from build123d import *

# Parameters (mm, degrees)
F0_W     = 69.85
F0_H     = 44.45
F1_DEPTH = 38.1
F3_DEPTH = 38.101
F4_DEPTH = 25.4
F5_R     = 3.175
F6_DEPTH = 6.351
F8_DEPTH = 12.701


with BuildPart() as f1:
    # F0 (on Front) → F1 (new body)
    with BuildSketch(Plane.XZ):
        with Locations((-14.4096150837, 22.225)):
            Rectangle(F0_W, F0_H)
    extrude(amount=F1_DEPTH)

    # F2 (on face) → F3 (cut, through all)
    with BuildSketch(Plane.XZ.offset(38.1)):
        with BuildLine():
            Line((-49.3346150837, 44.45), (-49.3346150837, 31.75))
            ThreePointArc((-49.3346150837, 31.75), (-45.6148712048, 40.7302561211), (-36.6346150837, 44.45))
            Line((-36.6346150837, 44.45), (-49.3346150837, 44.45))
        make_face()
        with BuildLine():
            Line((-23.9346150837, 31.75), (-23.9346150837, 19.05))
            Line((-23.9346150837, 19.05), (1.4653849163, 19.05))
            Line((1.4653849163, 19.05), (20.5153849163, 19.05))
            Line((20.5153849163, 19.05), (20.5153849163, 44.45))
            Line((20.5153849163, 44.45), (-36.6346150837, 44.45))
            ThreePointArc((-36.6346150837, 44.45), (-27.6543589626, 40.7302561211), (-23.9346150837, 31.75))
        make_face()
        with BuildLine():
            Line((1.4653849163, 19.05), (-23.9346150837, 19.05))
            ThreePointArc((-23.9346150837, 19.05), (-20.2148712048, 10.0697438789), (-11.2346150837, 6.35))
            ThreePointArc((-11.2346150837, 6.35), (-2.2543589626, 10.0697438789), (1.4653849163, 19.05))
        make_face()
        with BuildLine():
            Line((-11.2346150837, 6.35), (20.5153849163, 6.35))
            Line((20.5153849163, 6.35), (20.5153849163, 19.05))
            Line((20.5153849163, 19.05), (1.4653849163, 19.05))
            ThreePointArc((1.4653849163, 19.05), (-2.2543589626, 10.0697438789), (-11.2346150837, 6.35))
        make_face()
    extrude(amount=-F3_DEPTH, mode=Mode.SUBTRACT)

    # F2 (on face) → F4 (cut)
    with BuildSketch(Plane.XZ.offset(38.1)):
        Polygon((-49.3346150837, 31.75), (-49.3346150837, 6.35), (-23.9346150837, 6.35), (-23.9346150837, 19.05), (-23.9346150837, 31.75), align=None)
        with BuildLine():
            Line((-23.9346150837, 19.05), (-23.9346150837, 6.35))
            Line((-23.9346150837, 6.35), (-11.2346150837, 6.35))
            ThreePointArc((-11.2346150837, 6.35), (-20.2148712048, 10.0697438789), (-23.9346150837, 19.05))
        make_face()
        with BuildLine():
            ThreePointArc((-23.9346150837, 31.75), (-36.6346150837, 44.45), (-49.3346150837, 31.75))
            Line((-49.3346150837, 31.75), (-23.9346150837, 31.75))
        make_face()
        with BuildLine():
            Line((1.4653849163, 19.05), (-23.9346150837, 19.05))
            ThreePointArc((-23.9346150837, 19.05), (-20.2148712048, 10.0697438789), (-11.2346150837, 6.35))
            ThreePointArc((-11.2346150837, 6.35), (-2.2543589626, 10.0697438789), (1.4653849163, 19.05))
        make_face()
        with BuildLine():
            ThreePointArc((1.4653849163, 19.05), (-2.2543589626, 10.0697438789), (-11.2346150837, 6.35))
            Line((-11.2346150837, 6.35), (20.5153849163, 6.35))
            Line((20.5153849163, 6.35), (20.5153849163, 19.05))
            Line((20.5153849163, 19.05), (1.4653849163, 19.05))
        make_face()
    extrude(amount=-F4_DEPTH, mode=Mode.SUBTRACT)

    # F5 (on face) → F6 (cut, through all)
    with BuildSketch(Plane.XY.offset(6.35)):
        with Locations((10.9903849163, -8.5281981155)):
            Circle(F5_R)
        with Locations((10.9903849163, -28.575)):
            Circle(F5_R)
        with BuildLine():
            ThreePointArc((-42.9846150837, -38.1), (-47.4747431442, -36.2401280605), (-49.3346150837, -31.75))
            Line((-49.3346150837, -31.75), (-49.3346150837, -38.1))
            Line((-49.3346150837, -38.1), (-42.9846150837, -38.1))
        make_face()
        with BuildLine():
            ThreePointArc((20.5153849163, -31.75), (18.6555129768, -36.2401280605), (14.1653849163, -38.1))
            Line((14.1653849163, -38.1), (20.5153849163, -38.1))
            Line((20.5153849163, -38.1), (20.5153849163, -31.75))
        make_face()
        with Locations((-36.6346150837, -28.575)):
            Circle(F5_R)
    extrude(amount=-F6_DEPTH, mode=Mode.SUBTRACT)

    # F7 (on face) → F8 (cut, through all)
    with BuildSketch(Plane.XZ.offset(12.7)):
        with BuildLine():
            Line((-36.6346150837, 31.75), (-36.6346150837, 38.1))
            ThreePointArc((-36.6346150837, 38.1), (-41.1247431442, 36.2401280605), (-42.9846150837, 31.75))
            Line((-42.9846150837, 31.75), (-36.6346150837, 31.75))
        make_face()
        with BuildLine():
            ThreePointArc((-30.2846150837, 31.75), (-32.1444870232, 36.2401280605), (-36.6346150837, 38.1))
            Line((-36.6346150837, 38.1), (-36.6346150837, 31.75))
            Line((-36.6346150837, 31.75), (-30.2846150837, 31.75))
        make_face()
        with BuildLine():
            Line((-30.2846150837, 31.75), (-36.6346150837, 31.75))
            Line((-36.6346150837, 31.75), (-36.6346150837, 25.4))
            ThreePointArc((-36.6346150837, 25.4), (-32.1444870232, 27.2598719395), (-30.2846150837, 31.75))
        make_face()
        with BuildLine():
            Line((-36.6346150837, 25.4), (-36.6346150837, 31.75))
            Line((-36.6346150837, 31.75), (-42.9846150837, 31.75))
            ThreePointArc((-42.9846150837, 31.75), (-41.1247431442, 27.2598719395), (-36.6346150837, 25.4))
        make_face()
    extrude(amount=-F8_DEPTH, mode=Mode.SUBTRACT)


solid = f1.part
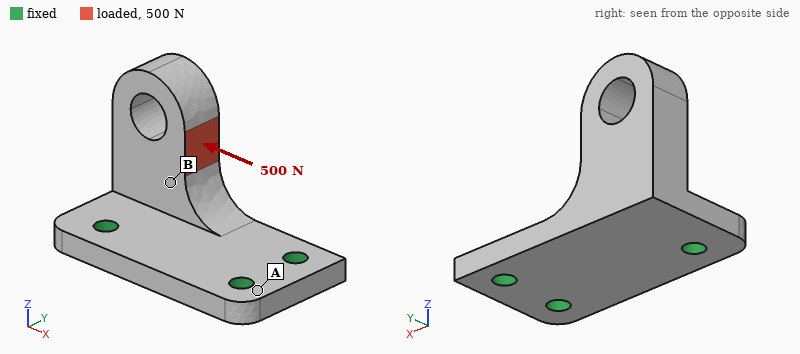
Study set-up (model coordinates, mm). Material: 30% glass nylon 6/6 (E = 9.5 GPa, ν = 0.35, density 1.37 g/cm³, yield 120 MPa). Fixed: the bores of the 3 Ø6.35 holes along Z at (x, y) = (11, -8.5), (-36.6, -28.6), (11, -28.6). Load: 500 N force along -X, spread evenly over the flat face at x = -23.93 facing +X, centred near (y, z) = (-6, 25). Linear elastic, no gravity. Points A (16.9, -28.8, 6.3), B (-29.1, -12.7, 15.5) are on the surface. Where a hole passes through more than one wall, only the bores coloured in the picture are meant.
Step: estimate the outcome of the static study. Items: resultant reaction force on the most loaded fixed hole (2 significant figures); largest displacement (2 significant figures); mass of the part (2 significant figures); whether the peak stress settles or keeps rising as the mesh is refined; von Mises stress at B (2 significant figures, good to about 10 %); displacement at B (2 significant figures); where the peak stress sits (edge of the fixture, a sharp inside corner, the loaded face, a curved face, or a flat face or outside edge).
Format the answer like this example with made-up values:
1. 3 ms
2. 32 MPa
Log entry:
1. 300 N
2. 0.33 mm
3. 36 g
4. keeps rising
5. 7.0 MPa
6. 0.093 mm
7. edge of the fixture
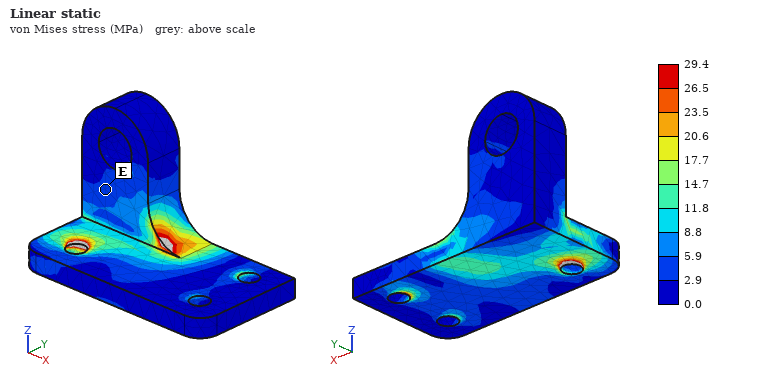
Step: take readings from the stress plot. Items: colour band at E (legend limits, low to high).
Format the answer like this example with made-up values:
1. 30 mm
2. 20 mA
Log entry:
1. 2.9 to 5.9 MPa
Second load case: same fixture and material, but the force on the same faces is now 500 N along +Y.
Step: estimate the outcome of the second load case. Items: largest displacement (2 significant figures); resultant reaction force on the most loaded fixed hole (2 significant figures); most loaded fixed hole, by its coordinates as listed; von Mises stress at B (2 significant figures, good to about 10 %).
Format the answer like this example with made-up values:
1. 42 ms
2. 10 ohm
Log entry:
1. 0.88 mm
2. 350 N
3. (-36.6, -28.6)
4. 14 MPa
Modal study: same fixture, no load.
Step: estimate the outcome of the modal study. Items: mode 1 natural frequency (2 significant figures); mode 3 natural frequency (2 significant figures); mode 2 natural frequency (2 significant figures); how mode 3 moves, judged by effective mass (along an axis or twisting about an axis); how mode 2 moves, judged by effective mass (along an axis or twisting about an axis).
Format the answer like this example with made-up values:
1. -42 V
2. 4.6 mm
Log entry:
1. 1200 Hz
2. 3800 Hz
3. 2300 Hz
4. along Z
5. along X
